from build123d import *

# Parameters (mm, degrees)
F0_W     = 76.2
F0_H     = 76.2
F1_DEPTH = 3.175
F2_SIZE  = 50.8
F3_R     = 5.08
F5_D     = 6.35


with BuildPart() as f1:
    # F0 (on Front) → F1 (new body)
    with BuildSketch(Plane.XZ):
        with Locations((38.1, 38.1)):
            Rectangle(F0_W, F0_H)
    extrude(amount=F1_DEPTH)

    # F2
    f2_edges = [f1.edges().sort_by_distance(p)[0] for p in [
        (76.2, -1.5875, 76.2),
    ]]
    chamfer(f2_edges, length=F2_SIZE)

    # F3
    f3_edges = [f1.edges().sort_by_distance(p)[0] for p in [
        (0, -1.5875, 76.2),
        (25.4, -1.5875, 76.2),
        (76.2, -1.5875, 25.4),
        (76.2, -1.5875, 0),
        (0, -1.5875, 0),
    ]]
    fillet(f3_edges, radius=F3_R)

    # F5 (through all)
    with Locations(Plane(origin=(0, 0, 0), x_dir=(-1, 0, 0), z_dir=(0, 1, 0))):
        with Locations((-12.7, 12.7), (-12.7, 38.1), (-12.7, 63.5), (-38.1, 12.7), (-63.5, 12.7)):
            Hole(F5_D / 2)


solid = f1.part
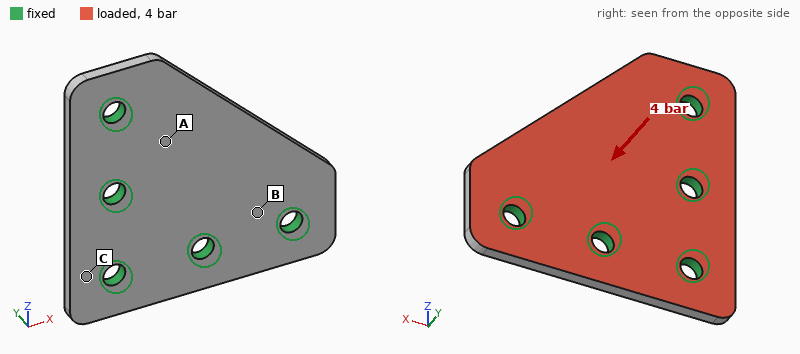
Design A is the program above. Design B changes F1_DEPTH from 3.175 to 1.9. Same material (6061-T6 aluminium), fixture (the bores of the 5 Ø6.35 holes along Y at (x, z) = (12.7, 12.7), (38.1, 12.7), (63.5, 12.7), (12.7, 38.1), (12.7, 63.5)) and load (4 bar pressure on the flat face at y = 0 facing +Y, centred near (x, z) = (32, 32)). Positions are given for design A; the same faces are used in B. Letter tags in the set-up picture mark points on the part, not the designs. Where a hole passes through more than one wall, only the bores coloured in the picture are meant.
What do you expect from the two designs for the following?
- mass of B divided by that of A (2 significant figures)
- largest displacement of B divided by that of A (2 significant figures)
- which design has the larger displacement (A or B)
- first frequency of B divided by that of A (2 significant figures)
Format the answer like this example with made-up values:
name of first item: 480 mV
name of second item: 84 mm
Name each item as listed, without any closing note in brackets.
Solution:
mass of B divided by that of A: 0.60
largest displacement of B divided by that of A: 4.5
which design has the larger displacement: B
first frequency of B divided by that of A: 0.61
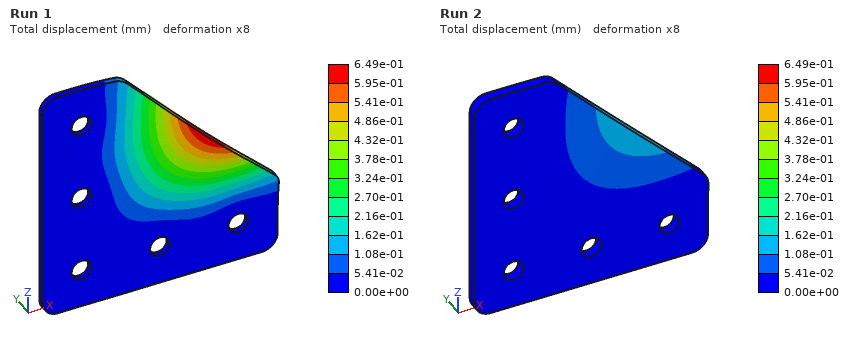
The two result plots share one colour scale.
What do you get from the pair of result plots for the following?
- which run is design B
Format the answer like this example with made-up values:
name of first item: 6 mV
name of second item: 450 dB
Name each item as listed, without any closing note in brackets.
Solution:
which run is design B: Run 1
